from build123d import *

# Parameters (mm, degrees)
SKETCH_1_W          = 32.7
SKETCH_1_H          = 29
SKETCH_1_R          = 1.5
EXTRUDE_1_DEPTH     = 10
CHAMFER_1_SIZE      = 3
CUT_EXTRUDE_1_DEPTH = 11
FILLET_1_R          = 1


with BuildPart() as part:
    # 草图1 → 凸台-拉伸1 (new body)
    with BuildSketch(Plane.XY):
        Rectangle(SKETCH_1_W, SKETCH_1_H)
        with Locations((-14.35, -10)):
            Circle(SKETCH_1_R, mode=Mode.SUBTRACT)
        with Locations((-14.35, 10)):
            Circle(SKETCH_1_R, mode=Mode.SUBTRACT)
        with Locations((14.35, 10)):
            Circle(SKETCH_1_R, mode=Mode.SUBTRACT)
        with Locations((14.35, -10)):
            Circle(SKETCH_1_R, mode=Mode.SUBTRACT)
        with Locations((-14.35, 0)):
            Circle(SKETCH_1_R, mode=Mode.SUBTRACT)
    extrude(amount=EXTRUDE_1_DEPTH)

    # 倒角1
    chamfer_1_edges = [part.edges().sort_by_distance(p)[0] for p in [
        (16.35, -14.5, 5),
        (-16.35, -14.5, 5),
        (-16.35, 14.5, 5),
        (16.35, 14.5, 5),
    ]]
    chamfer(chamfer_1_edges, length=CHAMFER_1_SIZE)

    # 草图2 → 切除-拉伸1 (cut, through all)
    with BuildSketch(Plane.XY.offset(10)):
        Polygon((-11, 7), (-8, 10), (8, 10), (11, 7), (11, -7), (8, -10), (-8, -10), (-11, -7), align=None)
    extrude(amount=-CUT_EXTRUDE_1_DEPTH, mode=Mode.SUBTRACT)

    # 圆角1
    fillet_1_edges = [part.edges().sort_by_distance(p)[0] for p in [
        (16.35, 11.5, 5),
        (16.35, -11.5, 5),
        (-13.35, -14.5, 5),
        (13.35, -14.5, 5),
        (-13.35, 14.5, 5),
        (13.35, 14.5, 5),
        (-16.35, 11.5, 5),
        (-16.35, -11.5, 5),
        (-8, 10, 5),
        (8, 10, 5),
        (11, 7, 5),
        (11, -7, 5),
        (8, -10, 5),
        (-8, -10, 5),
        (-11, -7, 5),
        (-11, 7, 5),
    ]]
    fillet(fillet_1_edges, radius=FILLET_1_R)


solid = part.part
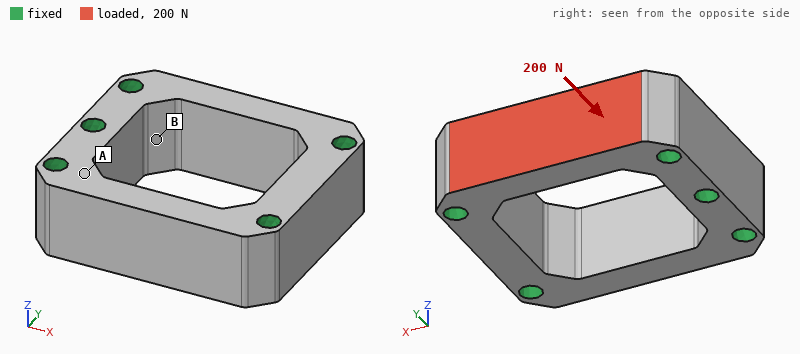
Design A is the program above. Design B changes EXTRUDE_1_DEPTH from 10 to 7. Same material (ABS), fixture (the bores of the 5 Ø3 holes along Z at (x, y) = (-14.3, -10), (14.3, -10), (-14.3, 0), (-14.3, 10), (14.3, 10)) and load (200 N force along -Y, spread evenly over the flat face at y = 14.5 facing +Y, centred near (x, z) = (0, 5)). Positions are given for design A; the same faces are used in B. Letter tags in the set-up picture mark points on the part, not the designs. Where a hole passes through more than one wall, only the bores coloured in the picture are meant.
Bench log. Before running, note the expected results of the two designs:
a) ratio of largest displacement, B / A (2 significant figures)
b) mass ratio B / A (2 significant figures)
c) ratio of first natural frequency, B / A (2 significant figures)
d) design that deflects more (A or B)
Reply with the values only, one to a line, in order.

1.4
0.70
0.99
B
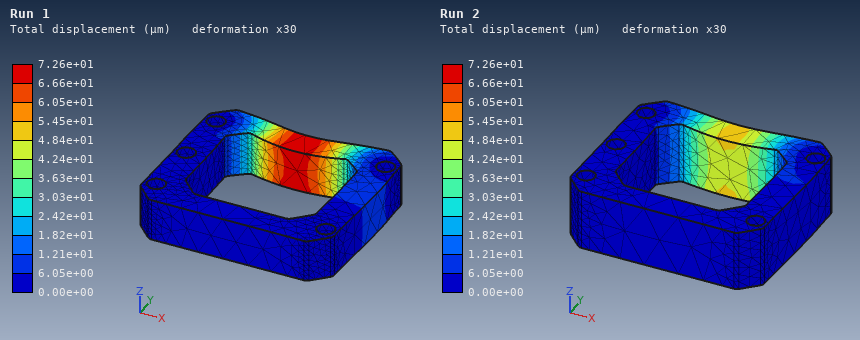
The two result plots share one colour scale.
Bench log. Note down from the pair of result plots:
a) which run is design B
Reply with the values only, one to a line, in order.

Run 1
